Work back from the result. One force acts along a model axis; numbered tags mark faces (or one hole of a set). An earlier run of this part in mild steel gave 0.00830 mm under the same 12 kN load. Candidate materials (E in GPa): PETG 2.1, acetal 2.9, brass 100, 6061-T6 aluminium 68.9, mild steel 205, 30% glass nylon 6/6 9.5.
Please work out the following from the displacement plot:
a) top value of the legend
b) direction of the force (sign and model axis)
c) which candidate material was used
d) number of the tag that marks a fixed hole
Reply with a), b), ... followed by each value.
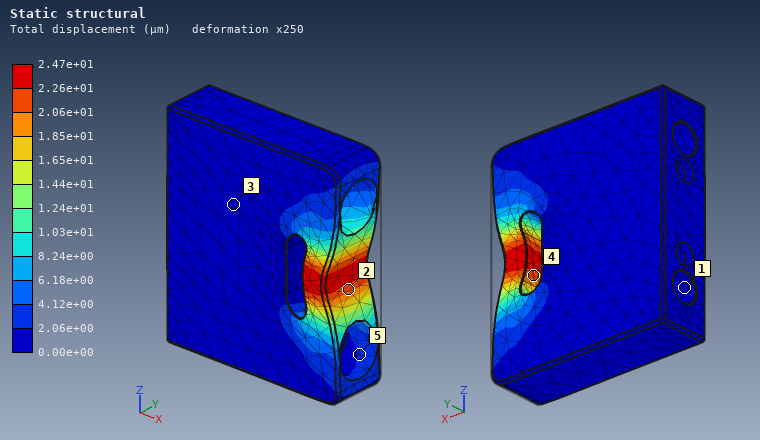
a) 2.47e+01 µm
b) -X
c) 6061-T6 aluminium
d) 1
